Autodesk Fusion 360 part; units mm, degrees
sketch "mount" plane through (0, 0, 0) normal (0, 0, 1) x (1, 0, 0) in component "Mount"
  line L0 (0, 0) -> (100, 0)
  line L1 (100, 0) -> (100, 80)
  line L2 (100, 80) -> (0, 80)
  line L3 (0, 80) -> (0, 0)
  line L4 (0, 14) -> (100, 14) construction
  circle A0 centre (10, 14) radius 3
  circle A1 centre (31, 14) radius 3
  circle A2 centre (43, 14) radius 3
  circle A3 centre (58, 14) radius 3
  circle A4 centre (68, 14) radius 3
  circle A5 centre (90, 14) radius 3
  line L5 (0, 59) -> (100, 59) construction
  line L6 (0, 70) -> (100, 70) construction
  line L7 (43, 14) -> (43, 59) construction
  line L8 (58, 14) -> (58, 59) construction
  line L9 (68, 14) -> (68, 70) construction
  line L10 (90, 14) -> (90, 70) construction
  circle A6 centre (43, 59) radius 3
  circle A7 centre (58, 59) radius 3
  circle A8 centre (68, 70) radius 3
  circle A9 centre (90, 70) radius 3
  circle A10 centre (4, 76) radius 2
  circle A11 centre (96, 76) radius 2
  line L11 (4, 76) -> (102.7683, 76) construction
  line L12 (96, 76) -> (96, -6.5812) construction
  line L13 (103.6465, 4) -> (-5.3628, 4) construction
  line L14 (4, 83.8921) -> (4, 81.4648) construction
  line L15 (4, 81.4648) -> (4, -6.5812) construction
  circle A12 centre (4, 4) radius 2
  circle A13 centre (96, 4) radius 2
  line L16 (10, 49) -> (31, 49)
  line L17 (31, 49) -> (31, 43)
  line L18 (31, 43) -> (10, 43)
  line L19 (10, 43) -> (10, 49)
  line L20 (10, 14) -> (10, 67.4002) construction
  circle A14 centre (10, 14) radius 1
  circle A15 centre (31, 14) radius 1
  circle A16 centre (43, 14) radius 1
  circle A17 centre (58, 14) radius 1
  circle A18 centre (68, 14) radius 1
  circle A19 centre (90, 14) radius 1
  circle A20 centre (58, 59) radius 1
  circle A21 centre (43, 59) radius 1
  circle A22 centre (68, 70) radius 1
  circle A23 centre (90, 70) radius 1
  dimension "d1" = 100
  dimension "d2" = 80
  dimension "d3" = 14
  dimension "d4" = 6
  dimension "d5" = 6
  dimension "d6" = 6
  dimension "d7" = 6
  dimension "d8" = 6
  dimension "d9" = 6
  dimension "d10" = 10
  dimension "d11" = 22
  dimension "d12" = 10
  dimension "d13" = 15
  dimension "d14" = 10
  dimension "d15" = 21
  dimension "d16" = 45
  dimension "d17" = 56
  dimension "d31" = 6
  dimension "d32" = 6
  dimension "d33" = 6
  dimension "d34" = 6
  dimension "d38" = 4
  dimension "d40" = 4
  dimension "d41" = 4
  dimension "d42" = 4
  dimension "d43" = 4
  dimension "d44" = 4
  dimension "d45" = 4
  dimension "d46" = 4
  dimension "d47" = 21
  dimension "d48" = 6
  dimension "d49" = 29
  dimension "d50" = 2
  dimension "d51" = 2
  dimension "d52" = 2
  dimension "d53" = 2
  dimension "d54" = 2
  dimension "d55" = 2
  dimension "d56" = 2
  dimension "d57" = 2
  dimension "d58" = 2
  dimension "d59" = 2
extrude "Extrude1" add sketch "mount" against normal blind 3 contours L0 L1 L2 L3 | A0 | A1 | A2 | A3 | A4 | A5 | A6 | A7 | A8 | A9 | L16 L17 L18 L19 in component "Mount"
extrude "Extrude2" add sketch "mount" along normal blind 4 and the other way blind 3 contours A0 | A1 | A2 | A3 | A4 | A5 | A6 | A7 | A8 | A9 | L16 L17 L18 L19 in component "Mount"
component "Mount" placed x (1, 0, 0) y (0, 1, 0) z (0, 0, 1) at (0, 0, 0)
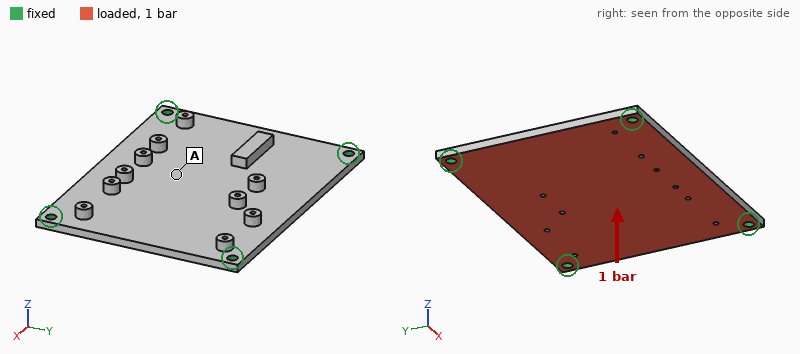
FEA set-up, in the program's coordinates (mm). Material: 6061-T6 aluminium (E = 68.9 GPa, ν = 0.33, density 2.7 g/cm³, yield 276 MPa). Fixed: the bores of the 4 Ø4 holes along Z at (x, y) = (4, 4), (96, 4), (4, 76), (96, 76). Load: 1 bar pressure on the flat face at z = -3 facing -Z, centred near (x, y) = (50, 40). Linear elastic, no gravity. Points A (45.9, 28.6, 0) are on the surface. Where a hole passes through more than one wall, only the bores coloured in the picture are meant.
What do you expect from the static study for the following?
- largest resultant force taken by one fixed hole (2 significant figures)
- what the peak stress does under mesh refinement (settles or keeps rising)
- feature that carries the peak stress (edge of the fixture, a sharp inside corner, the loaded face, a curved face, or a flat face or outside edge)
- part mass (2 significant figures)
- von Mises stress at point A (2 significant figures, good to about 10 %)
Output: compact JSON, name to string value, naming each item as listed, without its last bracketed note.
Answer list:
{"largest resultant force taken by one fixed hole": "200 N", "what the peak stress does under mesh refinement": "keeps rising", "feature that carries the peak stress": "edge of the fixture", "part mass": "68 g", "von Mises stress at point A": "27 MPa"}
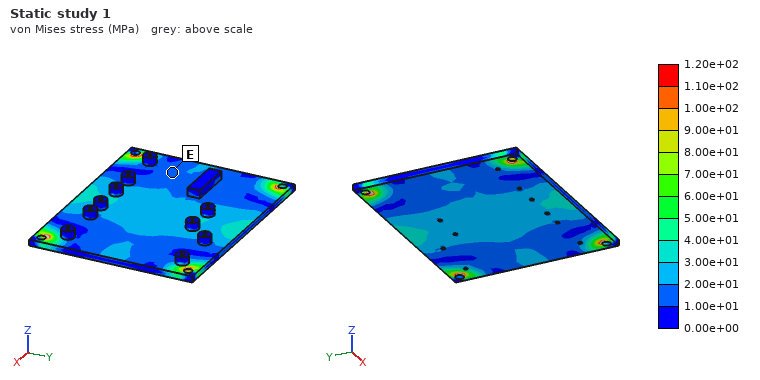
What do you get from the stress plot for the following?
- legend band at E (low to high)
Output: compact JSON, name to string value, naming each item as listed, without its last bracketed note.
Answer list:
{"legend band at E": "1.00e+01 to 2.00e+01 MPa"}
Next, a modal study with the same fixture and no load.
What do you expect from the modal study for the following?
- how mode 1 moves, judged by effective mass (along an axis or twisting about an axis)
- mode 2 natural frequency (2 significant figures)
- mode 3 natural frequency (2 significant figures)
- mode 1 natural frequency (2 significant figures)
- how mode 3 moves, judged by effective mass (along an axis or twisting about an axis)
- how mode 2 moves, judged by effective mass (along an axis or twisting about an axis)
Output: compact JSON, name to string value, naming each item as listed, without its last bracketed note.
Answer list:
{"how mode 1 moves, judged by effective mass": "along Z", "mode 2 natural frequency": "2200 Hz", "mode 3 natural frequency": "2900 Hz", "mode 1 natural frequency": "1300 Hz", "how mode 3 moves, judged by effective mass": "twisting about Y", "how mode 2 moves, judged by effective mass": "twisting about X"}
